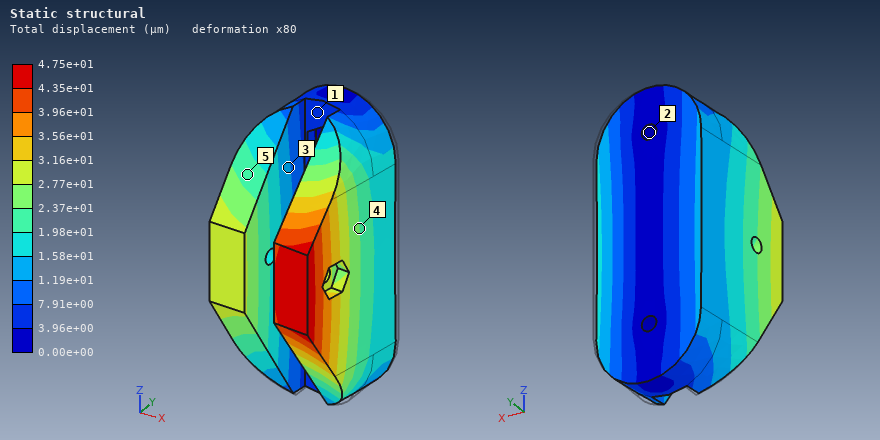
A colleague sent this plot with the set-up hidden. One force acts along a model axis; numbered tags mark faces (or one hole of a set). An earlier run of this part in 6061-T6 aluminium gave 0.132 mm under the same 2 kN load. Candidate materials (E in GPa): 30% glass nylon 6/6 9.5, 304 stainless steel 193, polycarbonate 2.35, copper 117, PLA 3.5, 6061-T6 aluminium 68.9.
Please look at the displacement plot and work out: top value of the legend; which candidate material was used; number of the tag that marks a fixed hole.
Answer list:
4.75e+01 µm
304 stainless steel
2
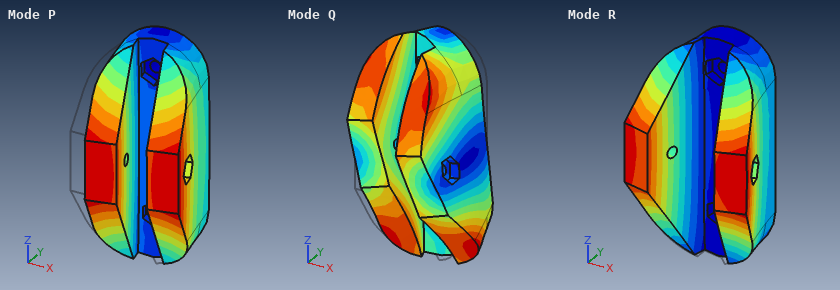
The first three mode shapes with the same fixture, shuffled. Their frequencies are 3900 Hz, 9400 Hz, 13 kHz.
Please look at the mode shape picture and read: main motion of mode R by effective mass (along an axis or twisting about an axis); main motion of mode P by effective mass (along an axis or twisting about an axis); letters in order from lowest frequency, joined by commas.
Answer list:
along Y
along X
P, R, Q
